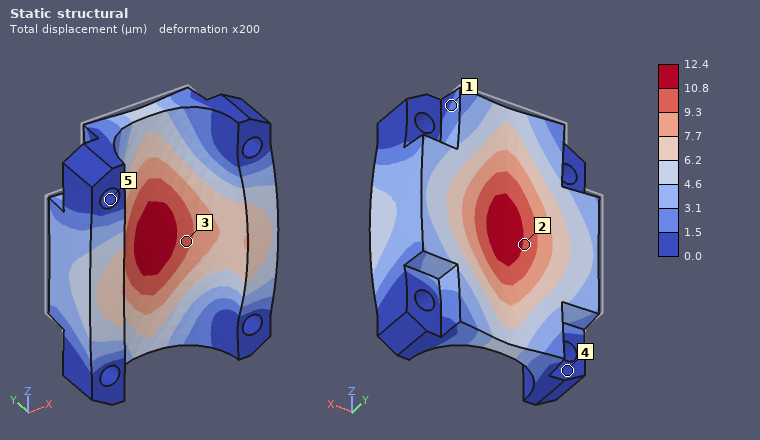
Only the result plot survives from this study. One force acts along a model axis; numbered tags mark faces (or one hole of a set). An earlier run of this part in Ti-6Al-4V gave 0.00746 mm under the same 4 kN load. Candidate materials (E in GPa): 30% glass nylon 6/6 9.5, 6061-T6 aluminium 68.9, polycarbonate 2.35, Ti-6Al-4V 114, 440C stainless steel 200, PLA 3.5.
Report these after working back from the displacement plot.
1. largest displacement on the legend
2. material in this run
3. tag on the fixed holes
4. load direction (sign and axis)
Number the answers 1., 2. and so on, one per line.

1. 12.4 µm
2. 6061-T6 aluminium
3. 5
4. -Y
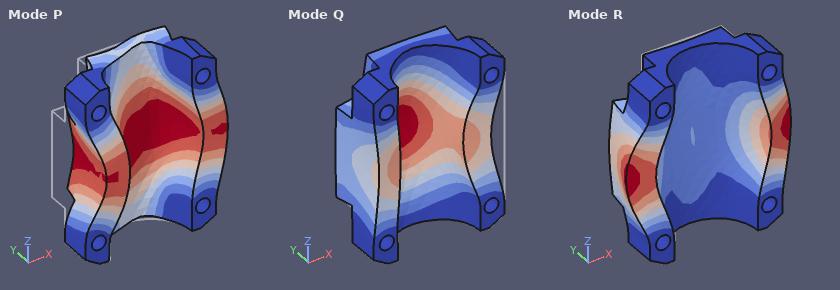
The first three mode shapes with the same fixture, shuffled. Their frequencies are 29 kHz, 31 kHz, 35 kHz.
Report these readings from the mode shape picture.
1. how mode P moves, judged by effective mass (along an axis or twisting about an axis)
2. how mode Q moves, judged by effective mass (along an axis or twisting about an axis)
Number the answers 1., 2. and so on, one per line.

1. along X
2. along Y
